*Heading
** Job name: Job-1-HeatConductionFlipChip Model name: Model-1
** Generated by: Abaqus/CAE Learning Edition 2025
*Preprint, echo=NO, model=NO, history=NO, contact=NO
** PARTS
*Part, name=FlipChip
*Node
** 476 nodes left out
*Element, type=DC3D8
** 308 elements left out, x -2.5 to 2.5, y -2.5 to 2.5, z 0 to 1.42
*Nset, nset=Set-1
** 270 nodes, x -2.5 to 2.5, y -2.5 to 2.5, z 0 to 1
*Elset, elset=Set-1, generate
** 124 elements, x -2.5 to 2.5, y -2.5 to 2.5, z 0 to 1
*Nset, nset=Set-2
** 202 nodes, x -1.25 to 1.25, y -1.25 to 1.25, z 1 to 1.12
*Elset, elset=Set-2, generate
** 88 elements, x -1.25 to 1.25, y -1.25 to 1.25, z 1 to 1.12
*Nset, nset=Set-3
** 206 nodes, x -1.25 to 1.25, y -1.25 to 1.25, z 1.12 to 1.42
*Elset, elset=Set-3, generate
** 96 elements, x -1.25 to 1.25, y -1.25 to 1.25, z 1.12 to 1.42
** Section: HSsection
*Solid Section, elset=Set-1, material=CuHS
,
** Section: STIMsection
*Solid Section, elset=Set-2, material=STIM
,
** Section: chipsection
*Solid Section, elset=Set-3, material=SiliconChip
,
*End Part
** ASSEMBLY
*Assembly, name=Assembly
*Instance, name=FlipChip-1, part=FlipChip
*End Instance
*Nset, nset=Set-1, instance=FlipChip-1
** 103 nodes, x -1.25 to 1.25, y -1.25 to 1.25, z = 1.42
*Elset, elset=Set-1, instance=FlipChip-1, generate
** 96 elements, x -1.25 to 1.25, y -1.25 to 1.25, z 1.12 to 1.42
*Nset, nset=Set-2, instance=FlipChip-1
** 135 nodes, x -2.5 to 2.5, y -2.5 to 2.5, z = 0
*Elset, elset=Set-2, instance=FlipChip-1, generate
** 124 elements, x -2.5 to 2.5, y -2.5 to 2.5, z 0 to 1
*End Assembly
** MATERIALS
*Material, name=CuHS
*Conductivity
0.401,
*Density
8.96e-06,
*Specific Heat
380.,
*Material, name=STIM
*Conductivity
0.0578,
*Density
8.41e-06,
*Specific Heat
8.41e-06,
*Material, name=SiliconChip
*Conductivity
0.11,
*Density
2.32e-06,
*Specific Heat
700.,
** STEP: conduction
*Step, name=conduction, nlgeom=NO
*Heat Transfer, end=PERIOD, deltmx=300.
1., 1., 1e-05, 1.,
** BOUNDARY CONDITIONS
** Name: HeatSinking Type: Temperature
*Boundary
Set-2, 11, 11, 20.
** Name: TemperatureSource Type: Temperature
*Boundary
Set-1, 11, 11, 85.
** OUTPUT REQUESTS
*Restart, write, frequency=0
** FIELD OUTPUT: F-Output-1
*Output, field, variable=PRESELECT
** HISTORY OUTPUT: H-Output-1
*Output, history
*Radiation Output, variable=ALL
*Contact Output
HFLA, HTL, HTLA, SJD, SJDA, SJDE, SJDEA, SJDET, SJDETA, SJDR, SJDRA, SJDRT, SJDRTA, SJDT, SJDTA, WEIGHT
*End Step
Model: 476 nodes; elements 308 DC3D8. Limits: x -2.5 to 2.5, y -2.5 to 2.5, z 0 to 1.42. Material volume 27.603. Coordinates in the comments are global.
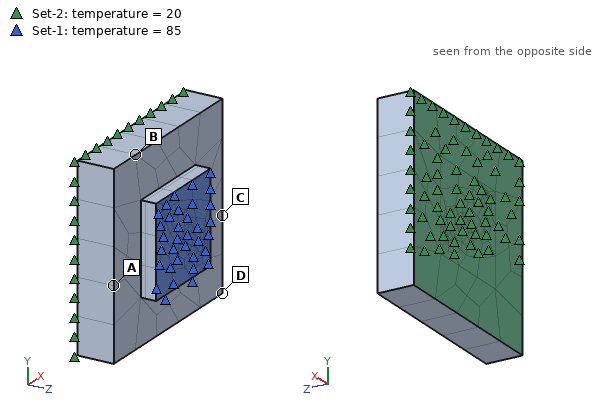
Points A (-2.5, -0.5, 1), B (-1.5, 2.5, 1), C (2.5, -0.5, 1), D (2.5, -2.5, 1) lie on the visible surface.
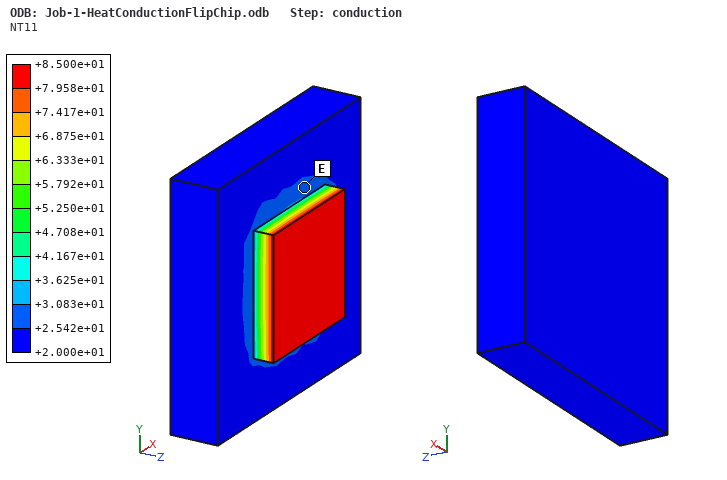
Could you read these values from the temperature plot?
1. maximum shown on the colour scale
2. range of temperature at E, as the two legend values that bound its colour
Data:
+8.500e+01
+2.542e+01 to +3.083e+01
